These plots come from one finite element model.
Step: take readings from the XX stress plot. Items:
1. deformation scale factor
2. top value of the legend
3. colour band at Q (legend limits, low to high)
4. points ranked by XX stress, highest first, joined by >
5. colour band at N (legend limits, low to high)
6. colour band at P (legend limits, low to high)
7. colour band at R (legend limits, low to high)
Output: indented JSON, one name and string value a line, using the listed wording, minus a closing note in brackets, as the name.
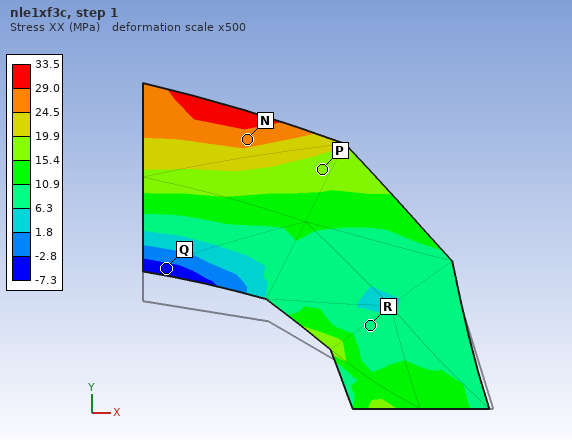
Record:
{
  "deformation scale factor": "500",
  "top value of the legend": "33.5 MPa",
  "colour band at Q": "-7.3 to -2.8 MPa",
  "points ranked by XX stress, highest first, joined by >": "N > P > R > Q",
  "colour band at N": "24.5 to 29.0 MPa",
  "colour band at P": "15.4 to 19.9 MPa",
  "colour band at R": "6.3 to 10.9 MPa"
}
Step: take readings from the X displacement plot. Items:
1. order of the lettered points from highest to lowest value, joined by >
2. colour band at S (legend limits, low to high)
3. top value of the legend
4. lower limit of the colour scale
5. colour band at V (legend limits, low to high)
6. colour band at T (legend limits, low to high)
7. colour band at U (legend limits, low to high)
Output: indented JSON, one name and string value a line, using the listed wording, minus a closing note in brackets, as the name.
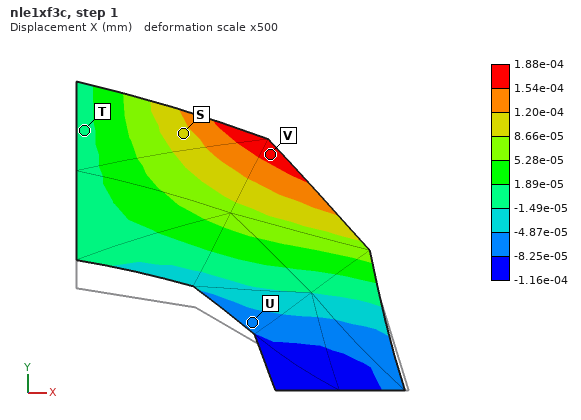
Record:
{
  "order of the lettered points from highest to lowest value, joined by >": "V > S > T > U",
  "colour band at S": "8.66e-05 to 1.20e-04 mm",
  "top value of the legend": "1.88e-04 mm",
  "lower limit of the colour scale": "-1.16e-04 mm",
  "colour band at V": "1.54e-04 to 1.88e-04 mm",
  "colour band at T": "-1.49e-05 to 1.89e-05 mm",
  "colour band at U": "-8.25e-05 to -4.87e-05 mm"
}
